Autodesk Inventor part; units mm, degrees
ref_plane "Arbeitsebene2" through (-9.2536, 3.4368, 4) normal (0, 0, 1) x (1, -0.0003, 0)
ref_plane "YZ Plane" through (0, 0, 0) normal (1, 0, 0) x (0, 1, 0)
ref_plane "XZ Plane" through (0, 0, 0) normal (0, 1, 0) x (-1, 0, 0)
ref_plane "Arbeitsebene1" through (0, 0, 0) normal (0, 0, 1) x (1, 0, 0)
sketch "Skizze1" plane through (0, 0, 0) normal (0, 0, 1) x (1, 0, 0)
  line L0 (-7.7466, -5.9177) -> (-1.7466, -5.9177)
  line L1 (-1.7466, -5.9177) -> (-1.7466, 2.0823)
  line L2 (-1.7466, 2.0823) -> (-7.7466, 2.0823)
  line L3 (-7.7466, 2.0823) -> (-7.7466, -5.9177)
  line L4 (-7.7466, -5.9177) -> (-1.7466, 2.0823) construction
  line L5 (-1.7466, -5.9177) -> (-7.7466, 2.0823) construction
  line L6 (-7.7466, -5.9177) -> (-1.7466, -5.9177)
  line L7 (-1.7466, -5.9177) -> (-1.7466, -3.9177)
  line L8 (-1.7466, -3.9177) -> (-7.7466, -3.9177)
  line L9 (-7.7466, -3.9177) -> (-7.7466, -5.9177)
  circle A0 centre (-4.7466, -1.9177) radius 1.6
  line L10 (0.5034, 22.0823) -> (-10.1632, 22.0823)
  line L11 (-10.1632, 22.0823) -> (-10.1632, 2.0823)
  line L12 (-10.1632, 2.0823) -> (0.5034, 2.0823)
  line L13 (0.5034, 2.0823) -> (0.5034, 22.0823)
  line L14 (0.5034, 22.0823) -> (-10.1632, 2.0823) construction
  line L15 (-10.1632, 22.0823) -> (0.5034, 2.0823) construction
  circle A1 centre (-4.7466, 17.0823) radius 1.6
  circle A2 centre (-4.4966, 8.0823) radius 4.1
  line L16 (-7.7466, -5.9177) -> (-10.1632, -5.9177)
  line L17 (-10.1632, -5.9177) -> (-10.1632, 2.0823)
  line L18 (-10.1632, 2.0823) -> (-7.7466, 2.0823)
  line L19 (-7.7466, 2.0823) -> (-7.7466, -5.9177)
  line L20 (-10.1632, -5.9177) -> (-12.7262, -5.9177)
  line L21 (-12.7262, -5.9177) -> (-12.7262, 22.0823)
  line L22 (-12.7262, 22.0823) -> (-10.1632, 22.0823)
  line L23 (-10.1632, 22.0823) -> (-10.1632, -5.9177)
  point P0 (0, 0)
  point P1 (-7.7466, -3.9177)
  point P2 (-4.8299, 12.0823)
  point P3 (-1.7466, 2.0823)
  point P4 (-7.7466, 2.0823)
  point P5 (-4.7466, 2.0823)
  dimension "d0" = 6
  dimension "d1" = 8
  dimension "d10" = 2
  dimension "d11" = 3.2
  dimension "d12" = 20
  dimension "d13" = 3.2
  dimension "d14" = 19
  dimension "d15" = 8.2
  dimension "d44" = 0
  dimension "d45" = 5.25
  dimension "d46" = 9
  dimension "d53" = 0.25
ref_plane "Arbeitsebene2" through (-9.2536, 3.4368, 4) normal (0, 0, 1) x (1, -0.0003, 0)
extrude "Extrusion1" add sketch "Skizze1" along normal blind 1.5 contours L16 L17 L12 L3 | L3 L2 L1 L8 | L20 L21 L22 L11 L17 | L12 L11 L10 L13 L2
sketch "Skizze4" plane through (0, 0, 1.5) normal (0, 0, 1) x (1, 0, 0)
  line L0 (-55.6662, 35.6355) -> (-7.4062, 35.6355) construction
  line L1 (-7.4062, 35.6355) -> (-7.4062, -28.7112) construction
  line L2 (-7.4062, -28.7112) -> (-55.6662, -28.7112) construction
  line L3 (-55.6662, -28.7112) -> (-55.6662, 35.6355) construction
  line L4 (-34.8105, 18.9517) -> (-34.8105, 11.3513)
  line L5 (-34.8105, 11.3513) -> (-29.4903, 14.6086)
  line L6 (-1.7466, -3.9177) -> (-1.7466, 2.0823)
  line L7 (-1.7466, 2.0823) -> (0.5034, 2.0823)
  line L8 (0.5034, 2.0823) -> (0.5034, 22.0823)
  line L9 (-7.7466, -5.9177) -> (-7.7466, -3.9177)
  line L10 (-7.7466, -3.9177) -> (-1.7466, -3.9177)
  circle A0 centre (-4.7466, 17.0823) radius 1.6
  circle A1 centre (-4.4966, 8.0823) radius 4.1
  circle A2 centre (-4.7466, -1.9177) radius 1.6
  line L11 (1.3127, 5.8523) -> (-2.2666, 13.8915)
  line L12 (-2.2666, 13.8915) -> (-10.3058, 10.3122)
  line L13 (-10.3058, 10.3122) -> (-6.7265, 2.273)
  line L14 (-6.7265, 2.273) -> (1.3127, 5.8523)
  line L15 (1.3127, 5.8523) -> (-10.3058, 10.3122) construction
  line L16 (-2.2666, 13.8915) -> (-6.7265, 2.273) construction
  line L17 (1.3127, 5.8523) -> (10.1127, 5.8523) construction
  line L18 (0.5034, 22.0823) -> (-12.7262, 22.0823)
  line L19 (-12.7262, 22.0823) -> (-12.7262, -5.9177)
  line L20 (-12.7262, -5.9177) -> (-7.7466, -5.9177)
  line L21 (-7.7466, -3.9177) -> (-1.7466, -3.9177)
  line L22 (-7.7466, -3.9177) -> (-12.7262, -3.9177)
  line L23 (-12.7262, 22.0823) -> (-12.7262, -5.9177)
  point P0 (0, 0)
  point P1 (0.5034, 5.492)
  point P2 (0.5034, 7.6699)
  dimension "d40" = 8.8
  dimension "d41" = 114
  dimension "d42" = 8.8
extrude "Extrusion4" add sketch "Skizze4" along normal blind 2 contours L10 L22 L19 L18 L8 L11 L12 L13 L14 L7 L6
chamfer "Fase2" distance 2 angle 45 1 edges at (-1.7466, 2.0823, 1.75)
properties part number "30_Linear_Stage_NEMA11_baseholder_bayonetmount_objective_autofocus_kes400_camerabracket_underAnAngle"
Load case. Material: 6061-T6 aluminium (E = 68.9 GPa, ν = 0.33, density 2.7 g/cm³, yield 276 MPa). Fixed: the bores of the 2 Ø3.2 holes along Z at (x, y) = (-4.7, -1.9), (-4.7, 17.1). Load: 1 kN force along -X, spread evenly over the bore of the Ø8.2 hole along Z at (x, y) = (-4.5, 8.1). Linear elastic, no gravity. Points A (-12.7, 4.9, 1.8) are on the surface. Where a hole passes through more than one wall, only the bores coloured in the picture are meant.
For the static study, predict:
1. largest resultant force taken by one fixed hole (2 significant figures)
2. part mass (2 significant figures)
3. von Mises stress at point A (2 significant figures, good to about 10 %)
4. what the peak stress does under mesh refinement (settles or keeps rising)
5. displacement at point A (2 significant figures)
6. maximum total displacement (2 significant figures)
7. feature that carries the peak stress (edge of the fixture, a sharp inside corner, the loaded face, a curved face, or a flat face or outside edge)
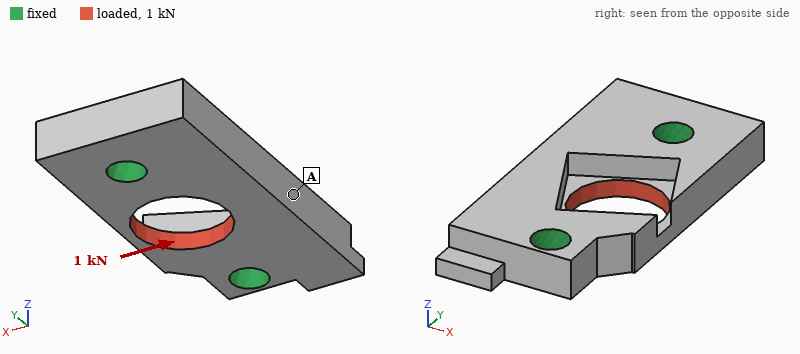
530 N
2.4 g
29 MPa
keeps rising
6.5 µm
23 µm
a sharp inside corner
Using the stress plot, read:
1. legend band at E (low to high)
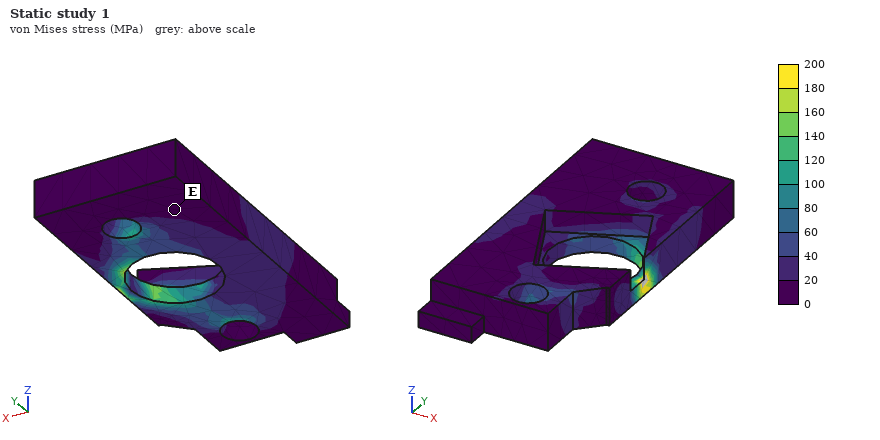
0 to 20 MPa
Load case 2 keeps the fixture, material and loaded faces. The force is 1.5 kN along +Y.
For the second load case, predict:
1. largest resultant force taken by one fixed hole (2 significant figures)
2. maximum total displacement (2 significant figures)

790 N
8.9 µm
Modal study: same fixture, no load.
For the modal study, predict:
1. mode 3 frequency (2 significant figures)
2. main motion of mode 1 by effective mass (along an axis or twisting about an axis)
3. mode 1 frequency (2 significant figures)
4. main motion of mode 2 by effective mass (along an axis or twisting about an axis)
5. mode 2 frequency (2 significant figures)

53 kHz
along Z
32 kHz
twisting about X
48 kHz
